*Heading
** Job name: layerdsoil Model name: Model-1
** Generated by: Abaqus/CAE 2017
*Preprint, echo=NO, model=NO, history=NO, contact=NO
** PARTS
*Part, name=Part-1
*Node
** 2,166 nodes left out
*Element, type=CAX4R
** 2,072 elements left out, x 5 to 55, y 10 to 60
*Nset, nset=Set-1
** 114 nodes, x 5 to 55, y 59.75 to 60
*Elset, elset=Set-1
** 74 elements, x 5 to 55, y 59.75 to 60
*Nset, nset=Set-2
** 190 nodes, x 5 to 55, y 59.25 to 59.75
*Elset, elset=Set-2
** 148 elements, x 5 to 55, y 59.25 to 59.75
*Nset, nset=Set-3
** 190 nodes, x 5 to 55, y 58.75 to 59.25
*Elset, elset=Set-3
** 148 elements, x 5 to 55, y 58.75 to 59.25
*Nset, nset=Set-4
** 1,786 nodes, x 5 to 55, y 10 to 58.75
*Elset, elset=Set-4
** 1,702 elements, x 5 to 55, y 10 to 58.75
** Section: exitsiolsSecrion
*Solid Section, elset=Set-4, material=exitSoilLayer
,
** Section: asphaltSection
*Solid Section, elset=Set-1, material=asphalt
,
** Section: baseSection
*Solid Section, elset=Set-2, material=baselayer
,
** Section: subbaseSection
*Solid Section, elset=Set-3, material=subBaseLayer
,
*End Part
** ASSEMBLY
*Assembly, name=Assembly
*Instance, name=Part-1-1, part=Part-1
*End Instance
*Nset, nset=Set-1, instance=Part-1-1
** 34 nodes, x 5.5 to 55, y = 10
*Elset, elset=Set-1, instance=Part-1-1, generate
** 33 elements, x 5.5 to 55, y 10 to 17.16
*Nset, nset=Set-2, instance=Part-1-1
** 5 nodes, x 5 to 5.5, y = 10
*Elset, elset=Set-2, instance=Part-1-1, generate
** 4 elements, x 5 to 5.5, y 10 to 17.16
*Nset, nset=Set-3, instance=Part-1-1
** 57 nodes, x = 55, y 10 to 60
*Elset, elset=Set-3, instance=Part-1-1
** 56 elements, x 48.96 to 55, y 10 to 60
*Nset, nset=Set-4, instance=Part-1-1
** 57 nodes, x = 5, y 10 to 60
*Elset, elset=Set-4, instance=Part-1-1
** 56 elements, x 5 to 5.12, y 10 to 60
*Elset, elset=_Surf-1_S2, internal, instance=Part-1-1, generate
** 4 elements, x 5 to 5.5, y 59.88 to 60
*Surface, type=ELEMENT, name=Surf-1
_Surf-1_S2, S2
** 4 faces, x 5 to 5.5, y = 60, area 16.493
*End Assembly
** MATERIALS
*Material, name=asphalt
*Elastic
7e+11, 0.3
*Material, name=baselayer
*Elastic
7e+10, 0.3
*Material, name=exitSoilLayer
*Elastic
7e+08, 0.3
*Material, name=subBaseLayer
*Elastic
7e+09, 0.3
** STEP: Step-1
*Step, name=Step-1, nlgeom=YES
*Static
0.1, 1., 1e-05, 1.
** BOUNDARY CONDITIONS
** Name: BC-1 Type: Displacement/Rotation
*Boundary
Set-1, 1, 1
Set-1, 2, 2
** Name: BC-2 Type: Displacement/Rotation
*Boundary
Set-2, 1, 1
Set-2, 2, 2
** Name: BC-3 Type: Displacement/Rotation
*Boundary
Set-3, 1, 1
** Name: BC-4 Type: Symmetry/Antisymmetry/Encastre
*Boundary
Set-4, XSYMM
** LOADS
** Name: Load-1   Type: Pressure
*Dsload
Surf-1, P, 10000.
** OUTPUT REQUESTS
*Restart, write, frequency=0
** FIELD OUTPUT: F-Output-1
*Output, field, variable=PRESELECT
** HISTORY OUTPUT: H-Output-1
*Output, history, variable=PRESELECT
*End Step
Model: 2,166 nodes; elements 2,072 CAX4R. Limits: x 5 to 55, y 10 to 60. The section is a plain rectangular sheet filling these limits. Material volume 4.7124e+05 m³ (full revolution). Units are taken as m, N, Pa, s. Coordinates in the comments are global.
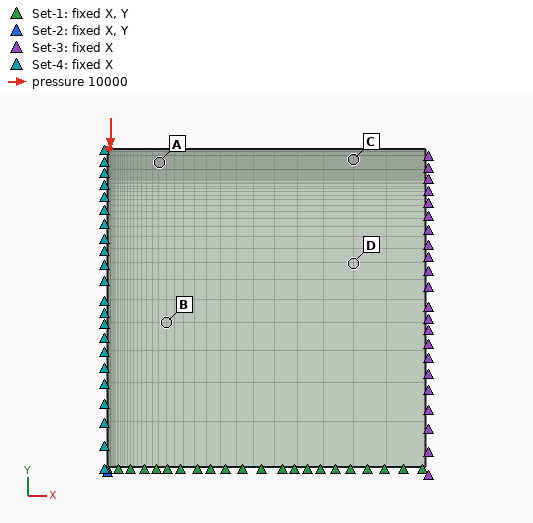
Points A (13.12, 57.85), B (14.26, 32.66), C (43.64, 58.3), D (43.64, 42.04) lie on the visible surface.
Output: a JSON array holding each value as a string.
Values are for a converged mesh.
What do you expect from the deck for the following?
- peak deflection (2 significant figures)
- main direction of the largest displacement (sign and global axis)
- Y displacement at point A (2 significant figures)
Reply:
["1.1e-05 m", "-Y", "-4.1e-06 m"]
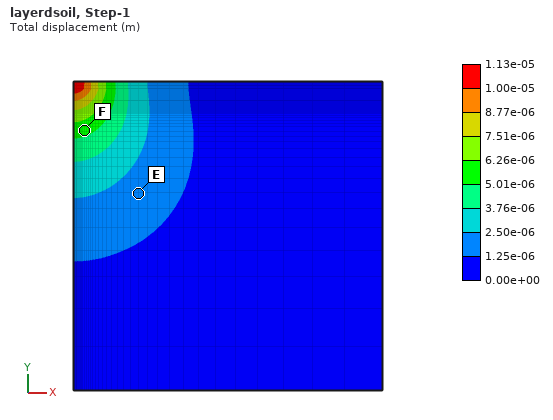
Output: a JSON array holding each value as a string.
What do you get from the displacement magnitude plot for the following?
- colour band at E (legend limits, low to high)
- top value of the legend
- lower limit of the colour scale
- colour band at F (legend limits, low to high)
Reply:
["1.25e-06 to 2.50e-06 m", "1.13e-05 m", "0.00e+00 m", "5.01e-06 to 6.26e-06 m"]
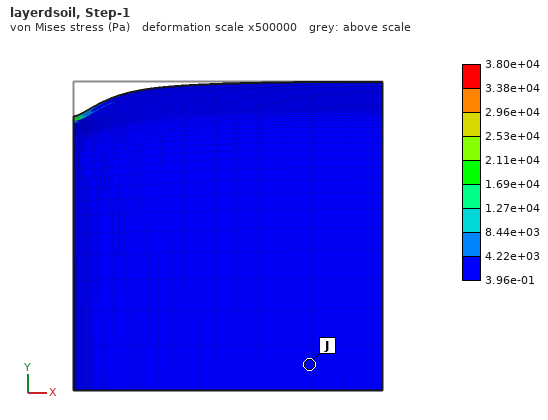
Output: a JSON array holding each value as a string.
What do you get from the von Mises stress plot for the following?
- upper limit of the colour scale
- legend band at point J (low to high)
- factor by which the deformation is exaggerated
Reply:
["3.80e+04 Pa", "3.96e-01 to 4.22e+03 Pa", "500000"]
